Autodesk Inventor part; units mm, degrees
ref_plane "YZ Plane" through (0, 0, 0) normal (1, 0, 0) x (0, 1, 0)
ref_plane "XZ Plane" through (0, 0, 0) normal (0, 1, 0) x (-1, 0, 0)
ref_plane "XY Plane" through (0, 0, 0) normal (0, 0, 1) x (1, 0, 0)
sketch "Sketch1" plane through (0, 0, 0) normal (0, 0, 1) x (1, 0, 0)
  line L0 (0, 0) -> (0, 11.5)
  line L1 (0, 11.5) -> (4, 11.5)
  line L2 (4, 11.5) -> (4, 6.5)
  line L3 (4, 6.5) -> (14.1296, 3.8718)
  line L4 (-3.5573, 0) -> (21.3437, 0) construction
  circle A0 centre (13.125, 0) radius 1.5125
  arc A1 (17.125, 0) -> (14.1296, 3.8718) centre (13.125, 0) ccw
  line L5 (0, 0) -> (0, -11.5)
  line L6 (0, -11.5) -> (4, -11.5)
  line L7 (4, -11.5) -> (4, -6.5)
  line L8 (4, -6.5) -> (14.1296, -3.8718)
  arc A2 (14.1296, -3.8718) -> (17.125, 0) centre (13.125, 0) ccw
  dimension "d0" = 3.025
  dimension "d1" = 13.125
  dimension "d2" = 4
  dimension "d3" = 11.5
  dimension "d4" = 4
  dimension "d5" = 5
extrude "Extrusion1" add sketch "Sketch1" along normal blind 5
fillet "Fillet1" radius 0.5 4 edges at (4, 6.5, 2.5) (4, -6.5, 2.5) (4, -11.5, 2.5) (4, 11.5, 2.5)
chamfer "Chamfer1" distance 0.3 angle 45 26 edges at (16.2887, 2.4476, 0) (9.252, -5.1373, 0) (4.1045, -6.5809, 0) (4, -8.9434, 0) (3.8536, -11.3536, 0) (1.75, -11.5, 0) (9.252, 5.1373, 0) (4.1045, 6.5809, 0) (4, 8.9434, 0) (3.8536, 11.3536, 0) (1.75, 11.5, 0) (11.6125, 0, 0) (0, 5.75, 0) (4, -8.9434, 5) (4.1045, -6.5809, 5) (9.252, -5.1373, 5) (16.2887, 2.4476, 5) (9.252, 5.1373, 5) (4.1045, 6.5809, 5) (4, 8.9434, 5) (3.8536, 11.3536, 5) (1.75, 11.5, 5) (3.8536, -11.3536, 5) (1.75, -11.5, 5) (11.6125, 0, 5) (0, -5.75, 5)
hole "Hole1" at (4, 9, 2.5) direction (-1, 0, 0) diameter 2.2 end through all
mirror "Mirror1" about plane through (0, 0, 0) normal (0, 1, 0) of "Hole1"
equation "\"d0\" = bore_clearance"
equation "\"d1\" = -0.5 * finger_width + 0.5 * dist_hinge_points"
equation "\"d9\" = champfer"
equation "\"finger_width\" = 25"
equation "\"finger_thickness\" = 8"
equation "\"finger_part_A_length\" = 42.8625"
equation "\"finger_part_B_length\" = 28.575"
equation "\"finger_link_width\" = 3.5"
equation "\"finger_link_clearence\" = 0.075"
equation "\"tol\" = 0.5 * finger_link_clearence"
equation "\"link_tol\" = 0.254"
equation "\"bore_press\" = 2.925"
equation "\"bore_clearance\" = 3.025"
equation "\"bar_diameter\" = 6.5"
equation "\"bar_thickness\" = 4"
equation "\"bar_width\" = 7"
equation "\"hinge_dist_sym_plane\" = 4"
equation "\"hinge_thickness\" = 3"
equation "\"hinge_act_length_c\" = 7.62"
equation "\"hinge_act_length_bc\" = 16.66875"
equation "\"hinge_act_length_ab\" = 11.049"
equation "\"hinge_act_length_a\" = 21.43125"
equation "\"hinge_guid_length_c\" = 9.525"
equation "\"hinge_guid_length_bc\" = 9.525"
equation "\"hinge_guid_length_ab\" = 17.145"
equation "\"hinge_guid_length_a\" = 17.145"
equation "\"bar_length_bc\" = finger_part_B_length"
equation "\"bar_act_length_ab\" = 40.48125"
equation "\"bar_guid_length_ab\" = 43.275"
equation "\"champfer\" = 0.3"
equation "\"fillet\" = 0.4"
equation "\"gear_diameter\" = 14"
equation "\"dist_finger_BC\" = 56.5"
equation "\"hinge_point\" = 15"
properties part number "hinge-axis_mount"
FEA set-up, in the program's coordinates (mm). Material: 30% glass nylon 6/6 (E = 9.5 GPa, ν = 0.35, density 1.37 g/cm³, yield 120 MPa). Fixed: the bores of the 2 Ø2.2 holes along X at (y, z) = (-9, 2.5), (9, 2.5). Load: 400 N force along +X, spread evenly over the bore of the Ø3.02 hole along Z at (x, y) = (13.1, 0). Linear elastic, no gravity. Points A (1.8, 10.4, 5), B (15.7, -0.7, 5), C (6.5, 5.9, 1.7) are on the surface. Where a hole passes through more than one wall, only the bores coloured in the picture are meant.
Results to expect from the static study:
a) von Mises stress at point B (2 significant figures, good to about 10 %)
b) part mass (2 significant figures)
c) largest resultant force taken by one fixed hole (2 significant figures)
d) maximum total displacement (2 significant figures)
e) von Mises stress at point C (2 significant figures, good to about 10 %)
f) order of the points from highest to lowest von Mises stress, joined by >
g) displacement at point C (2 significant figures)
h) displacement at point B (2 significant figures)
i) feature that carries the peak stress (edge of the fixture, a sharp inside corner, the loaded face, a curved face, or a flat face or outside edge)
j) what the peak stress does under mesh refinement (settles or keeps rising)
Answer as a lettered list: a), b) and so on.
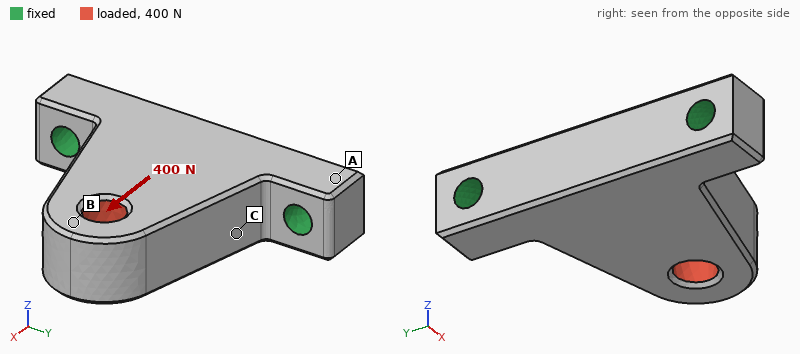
a) 7.2 MPa
b) 1.4 g
c) 220 N
d) 28 µm
e) 14 MPa
f) C > B > A
g) 16 µm
h) 27 µm
i) edge of the fixture
j) keeps rising
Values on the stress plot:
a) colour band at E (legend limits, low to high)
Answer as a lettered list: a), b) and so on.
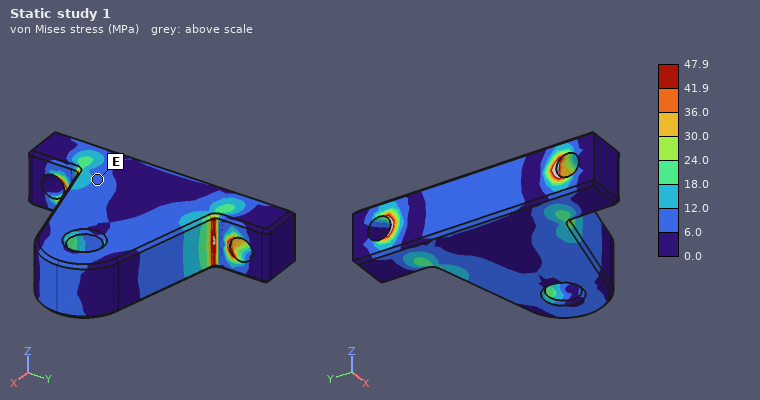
a) 6.0 to 12.0 MPa
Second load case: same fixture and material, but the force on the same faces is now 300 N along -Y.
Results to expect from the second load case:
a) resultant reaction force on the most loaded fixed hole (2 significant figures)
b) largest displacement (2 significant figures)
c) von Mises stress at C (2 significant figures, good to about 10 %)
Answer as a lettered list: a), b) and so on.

a) 270 N
b) 70 µm
c) 23 MPa
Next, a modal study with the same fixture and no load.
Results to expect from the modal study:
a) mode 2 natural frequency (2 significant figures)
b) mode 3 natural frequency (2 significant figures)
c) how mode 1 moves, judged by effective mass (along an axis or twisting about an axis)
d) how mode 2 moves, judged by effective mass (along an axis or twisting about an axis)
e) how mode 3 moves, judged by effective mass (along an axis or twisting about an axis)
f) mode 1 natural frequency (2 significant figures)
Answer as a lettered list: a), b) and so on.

a) 19 kHz
b) 23 kHz
c) along Z
d) along Y
e) along X
f) 6400 Hz
